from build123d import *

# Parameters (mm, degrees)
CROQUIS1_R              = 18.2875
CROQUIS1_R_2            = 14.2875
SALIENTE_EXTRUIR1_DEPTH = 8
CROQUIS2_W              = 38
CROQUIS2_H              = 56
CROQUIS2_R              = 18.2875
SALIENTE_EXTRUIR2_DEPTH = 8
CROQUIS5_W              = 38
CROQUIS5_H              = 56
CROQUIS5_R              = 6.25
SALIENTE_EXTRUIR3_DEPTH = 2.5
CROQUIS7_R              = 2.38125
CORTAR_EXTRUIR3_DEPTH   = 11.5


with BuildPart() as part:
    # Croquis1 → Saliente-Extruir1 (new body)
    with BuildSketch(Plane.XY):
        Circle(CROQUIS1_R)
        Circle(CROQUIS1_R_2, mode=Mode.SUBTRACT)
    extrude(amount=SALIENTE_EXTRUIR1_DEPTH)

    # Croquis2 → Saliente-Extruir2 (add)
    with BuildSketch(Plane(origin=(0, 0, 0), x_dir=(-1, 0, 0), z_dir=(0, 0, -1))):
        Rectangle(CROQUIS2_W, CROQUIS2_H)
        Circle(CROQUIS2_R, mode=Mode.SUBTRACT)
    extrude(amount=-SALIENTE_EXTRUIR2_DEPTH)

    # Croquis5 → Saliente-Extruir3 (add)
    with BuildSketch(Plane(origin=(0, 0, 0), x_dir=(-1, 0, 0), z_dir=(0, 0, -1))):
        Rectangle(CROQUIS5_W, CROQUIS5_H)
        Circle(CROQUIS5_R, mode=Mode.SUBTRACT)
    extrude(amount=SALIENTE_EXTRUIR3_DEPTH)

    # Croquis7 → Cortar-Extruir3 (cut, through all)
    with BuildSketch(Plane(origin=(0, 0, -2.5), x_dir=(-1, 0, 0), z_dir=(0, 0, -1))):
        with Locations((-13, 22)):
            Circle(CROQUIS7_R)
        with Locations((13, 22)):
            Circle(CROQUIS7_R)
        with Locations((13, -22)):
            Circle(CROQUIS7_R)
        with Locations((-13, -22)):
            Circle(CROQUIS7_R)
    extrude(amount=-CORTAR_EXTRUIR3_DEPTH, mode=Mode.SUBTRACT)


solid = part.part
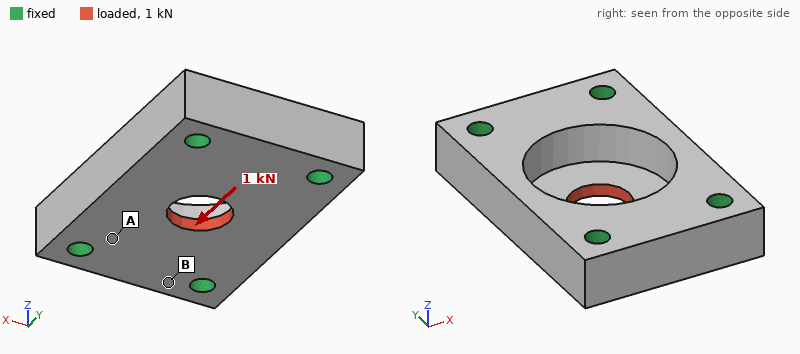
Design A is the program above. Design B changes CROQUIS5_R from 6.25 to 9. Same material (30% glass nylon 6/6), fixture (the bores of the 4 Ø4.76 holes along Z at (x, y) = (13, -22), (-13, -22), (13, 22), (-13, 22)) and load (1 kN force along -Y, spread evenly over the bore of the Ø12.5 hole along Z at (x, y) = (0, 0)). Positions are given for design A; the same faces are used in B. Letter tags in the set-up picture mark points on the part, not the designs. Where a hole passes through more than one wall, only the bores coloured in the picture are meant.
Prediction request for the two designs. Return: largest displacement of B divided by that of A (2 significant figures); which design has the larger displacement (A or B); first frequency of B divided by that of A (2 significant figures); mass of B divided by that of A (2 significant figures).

0.83
A
1.1
0.98
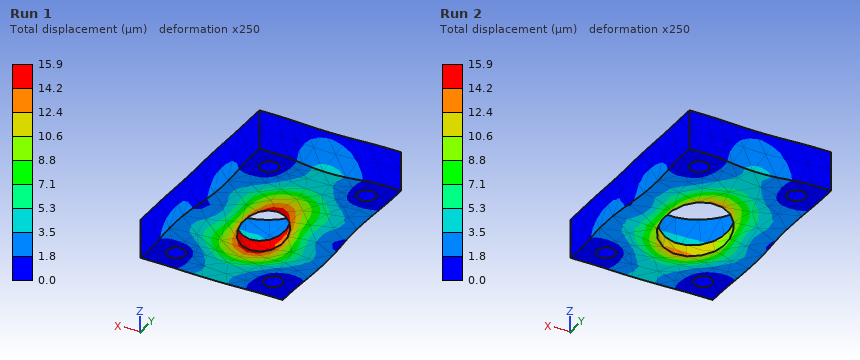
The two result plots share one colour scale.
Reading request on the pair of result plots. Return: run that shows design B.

Run 2
